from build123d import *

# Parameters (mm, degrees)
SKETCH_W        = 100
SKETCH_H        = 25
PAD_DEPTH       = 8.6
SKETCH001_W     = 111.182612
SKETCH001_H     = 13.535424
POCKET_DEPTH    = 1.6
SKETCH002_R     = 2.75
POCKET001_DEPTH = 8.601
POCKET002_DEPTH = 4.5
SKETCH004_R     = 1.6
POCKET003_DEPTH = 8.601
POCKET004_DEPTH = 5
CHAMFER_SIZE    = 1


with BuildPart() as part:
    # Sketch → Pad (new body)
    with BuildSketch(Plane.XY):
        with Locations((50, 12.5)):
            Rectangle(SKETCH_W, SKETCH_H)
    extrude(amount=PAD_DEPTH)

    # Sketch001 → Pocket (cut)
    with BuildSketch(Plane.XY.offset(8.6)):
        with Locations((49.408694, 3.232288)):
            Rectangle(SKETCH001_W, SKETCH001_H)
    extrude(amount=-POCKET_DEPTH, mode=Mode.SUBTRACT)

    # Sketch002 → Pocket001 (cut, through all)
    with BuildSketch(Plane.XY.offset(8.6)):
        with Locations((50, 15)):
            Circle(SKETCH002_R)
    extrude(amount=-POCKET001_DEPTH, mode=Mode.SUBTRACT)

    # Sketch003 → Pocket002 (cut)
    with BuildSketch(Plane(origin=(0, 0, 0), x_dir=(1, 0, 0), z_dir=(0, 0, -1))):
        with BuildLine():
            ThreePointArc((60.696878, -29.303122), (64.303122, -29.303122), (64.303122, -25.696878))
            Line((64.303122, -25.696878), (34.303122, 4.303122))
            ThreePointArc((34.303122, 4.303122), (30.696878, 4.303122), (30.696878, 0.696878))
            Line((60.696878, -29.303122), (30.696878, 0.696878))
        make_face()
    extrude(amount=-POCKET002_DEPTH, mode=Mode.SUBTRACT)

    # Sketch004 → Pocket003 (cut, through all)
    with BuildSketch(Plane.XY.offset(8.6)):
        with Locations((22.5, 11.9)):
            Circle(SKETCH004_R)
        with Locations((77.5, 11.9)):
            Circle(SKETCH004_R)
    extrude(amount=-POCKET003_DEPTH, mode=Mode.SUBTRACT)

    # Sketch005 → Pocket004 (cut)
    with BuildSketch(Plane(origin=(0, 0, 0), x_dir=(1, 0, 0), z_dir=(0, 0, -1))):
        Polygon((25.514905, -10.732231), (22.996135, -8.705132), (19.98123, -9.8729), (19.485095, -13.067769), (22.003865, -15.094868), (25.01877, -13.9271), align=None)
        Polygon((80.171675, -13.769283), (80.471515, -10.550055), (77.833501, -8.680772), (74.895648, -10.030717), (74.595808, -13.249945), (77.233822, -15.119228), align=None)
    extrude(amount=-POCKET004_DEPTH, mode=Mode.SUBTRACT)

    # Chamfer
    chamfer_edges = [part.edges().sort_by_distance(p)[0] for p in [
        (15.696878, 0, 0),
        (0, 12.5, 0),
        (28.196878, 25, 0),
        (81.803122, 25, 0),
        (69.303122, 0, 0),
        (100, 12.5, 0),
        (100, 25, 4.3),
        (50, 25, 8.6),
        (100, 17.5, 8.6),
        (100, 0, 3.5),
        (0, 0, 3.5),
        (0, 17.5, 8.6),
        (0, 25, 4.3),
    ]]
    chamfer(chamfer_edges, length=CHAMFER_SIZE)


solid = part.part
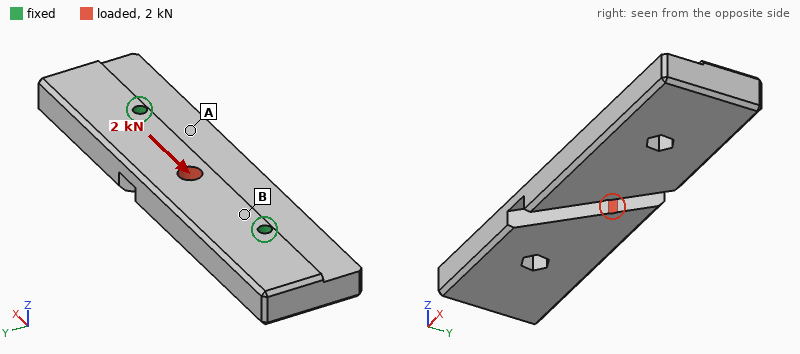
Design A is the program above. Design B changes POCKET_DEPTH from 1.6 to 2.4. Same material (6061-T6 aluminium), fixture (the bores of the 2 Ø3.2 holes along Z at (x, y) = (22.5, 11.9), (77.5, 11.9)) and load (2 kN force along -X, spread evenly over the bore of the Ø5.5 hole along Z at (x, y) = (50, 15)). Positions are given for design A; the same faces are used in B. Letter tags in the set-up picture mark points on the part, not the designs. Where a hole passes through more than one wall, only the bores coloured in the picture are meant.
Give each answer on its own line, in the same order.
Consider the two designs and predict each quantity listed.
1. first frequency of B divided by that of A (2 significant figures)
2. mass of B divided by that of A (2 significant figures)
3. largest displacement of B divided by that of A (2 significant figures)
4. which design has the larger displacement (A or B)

0.98
0.96
1.1
B
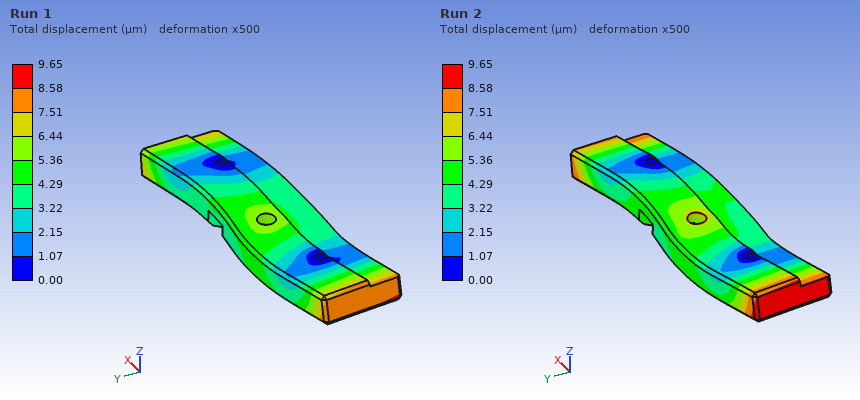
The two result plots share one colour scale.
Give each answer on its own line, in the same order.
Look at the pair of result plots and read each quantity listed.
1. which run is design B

Run 2
